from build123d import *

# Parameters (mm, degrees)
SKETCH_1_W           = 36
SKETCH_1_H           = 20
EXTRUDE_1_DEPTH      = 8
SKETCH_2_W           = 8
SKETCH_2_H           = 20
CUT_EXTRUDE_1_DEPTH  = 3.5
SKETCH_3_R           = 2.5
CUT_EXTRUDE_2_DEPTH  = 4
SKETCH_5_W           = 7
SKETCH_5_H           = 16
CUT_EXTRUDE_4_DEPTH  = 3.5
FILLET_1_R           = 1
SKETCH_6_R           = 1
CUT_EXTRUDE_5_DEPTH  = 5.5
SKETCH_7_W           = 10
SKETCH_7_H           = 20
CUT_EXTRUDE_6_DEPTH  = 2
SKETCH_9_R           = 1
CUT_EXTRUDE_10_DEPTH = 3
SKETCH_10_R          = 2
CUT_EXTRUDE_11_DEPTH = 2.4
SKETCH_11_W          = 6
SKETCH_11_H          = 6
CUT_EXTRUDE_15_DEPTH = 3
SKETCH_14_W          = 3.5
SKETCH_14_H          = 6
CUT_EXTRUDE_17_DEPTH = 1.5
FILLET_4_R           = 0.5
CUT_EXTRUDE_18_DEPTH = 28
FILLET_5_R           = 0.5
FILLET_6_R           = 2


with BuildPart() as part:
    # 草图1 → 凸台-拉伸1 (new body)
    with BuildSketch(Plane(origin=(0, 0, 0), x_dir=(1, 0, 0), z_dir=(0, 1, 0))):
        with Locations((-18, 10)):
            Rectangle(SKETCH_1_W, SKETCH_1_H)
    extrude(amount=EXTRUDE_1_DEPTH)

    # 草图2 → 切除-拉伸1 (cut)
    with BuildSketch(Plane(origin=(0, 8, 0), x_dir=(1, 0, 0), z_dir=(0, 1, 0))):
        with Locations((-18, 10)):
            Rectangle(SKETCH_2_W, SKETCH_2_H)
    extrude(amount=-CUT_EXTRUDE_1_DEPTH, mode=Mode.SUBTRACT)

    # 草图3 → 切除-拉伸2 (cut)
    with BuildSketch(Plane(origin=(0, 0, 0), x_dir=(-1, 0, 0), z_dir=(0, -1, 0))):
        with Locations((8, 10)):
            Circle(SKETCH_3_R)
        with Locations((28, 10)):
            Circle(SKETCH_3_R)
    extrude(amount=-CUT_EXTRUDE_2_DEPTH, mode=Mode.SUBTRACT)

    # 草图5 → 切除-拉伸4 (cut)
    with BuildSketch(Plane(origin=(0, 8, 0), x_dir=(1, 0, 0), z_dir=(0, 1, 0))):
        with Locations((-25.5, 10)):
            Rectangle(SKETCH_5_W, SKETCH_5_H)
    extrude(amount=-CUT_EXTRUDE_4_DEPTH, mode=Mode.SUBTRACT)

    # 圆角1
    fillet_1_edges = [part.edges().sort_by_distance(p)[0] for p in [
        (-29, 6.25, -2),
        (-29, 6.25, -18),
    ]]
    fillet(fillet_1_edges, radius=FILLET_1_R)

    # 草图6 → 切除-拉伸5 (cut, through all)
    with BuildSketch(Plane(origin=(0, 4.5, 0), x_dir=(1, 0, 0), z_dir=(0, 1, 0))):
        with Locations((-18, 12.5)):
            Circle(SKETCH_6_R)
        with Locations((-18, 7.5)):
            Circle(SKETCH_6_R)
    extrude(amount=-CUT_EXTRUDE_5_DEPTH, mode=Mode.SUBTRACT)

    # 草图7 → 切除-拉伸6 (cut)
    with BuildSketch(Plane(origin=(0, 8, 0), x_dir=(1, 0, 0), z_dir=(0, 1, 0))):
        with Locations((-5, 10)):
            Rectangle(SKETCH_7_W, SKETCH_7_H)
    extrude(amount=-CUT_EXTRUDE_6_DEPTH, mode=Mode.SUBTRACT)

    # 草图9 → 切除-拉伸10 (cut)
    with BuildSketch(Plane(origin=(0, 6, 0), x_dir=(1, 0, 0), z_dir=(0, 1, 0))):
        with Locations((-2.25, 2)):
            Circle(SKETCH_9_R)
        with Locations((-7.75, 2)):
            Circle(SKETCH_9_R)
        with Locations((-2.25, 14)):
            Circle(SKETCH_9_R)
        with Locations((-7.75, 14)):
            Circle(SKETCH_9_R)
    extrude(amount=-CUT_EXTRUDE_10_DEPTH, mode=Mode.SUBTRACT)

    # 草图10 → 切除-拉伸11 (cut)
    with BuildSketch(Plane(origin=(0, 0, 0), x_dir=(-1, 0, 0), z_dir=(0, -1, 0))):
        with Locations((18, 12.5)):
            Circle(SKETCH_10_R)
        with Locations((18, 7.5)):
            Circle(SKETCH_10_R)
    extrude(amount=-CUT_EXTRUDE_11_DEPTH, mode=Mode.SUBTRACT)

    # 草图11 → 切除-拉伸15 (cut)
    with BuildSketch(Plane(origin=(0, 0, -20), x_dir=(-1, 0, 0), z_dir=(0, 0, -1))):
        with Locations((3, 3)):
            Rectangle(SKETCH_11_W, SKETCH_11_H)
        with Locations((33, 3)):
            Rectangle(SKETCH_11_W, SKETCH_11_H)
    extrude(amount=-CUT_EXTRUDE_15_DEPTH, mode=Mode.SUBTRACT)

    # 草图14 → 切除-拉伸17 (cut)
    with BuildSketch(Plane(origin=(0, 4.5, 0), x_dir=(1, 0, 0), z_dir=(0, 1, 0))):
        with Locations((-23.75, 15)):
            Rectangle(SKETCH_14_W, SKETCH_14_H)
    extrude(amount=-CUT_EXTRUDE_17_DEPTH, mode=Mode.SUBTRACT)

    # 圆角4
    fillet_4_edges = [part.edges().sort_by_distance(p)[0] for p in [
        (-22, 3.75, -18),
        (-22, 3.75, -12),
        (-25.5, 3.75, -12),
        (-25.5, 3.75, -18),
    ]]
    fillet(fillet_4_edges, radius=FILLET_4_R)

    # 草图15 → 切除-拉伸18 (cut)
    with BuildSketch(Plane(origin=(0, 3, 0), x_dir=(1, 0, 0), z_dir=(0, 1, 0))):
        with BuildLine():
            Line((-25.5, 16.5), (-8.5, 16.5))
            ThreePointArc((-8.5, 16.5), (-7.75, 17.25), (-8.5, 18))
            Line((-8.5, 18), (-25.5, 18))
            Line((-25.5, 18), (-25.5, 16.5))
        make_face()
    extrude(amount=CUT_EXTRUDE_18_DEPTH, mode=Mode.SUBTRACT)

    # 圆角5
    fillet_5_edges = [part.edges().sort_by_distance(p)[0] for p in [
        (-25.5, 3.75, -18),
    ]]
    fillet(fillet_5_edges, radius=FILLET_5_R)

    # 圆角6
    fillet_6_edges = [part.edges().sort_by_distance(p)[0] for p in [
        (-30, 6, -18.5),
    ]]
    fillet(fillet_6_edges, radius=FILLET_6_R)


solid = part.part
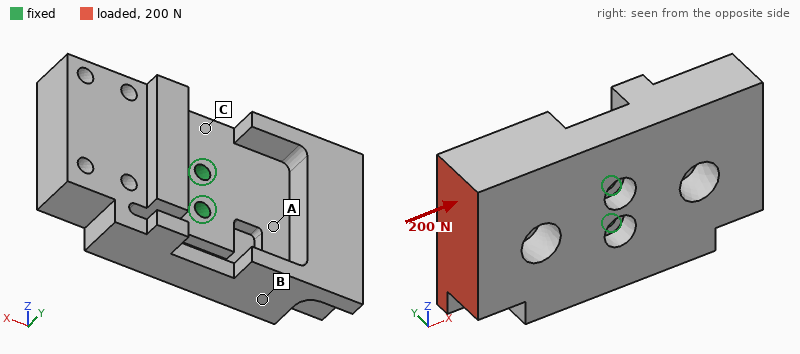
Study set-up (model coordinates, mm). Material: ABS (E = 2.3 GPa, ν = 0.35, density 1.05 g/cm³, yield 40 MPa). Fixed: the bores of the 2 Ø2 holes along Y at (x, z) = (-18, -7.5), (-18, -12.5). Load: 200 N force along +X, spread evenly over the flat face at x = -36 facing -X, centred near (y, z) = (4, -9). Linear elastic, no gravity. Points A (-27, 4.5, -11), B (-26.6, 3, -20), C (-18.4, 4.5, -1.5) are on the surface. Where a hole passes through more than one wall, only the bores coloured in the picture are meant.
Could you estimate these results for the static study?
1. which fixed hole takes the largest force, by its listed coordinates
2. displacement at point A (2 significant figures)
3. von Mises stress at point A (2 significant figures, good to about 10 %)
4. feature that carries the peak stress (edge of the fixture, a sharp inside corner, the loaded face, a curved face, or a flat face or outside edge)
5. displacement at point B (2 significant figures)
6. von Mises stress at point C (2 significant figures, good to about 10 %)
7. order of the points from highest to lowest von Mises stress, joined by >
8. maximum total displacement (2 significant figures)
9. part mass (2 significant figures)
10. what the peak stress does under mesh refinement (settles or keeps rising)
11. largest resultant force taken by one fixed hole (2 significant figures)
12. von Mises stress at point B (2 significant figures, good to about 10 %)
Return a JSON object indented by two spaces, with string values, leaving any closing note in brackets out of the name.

{
  "which fixed hole takes the largest force, by its listed coordinates": "(-18, -7.5)",
  "displacement at point A": "0.082 mm",
  "von Mises stress at point A": "12 MPa",
  "feature that carries the peak stress": "edge of the fixture",
  "displacement at point B": "0.072 mm",
  "von Mises stress at point C": "5.9 MPa",
  "order of the points from highest to lowest von Mises stress, joined by >": "A > C > B",
  "maximum total displacement": "0.24 mm",
  "part mass": "4.0 g",
  "what the peak stress does under mesh refinement": "keeps rising",
  "largest resultant force taken by one fixed hole": "140 N",
  "von Mises stress at point B": "1.6 MPa"
}
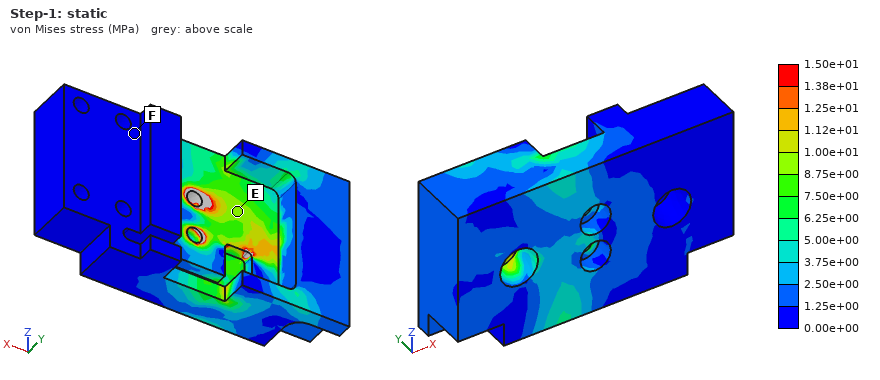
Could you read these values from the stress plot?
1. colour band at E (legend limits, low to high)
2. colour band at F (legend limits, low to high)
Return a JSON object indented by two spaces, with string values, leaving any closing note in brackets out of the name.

{
  "colour band at E": "8.75e+00 to 1.00e+01 MPa",
  "colour band at F": "0.00e+00 to 1.25e+00 MPa"
}
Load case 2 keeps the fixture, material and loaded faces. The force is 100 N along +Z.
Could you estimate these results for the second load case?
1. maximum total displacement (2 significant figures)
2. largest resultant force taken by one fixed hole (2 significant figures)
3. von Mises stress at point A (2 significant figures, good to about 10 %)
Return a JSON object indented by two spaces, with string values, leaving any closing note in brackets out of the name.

{
  "maximum total displacement": "0.27 mm",
  "largest resultant force taken by one fixed hole": "280 N",
  "von Mises stress at point A": "6.9 MPa"
}
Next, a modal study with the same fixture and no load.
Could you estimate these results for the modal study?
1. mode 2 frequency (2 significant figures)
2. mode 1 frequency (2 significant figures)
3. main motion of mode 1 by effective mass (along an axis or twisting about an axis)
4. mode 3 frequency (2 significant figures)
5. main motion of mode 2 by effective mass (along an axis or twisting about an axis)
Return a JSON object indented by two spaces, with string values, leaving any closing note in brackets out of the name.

{
  "mode 2 frequency": "2600 Hz",
  "mode 1 frequency": "1200 Hz",
  "main motion of mode 1 by effective mass": "twisting about Z",
  "mode 3 frequency": "2700 Hz",
  "main motion of mode 2 by effective mass": "along Y"
}
